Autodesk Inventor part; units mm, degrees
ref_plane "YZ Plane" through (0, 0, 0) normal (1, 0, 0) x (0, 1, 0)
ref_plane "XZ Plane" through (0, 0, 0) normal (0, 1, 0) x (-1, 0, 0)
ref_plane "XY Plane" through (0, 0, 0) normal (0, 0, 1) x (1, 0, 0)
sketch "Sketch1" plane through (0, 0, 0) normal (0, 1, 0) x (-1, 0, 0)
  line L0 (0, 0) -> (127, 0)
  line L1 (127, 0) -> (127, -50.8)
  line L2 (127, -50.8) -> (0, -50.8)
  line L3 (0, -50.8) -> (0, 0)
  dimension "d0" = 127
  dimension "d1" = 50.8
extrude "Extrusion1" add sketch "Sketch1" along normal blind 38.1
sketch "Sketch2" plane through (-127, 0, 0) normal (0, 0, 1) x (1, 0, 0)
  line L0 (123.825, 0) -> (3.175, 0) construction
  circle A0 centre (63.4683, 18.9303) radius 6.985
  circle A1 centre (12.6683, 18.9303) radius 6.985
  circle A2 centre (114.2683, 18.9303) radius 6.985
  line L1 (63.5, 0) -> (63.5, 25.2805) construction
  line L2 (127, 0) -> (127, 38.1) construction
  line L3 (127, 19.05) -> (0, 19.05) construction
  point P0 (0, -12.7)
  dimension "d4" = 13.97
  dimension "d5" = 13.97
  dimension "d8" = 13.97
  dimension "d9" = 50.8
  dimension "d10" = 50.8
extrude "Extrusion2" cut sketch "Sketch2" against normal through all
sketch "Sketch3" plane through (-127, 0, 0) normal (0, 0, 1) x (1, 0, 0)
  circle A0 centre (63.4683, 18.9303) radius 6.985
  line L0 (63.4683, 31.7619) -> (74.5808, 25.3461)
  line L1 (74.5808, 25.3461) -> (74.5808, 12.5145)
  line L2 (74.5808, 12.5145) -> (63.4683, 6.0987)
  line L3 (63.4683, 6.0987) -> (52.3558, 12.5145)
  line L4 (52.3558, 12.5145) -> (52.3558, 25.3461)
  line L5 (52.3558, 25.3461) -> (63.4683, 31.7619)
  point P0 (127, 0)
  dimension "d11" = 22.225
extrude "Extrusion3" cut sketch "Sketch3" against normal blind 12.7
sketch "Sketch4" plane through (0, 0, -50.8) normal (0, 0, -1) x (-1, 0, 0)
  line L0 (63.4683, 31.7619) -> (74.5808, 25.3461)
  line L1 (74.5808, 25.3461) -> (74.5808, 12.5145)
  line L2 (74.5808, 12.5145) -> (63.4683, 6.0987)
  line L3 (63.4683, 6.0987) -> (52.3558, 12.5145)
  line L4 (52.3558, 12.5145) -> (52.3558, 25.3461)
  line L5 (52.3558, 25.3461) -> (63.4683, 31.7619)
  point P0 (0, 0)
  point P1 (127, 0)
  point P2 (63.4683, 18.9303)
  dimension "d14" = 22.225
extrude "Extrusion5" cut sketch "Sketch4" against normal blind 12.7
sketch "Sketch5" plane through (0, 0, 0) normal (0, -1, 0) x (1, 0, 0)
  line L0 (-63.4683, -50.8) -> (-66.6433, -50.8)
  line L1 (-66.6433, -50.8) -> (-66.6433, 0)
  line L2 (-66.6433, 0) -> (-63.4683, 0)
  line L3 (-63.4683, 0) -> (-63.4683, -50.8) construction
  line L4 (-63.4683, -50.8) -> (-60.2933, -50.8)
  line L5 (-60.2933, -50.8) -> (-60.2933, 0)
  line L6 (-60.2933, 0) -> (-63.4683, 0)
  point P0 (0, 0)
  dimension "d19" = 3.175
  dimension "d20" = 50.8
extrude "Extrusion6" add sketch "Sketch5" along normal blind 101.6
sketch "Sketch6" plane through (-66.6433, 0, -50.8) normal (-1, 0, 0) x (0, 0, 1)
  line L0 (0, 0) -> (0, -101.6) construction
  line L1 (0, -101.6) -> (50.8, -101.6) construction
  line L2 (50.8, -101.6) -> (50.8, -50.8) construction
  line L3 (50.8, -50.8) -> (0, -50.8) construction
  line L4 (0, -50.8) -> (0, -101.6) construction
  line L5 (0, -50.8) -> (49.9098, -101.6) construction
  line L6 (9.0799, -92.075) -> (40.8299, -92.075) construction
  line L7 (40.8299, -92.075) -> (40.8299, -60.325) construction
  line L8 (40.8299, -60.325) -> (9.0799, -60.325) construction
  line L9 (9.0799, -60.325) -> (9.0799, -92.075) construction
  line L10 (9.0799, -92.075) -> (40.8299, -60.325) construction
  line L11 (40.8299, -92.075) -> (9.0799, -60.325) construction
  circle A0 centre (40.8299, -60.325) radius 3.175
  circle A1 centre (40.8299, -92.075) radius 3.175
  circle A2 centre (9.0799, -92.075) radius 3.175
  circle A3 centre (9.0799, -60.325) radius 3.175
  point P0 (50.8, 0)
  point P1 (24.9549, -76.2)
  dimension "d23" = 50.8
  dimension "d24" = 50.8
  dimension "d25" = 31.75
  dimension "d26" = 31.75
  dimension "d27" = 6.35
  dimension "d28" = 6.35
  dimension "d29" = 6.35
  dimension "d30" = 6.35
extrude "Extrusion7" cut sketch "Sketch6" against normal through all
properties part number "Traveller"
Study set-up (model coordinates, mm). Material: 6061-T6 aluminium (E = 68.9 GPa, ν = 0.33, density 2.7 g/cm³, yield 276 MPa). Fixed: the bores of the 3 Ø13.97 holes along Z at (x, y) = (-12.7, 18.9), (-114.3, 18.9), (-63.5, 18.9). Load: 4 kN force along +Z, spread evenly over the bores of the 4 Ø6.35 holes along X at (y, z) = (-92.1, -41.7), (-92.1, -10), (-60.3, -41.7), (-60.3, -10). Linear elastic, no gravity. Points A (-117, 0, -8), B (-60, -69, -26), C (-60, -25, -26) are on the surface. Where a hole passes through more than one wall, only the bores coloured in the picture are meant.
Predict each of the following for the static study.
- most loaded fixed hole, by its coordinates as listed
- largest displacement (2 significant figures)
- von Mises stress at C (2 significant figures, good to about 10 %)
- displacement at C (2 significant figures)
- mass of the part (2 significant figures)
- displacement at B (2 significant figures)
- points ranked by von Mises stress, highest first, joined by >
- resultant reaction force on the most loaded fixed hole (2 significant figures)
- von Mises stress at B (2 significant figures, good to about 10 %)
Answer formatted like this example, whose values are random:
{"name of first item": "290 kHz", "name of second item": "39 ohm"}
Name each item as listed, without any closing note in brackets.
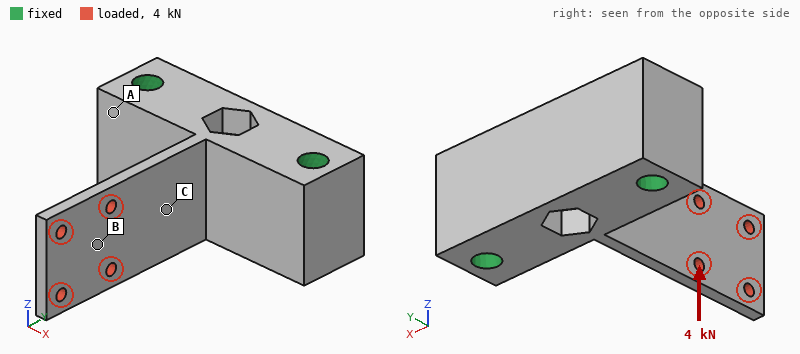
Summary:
{"most loaded fixed hole, by its coordinates as listed": "(-63.5, 18.9)", "largest displacement": "0.38 mm", "von Mises stress at C": "33 MPa", "displacement at C": "0.072 mm", "mass of the part": "670 g", "displacement at B": "0.24 mm", "points ranked by von Mises stress, highest first, joined by >": "C > B > A", "resultant reaction force on the most loaded fixed hole": "4.1 kN", "von Mises stress at B": "19 MPa"}
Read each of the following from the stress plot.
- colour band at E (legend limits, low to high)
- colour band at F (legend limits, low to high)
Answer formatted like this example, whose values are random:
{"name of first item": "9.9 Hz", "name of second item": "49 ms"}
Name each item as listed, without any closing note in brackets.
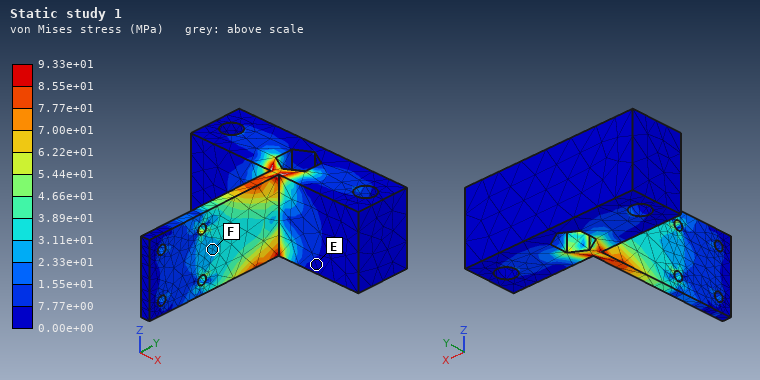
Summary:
{"colour band at E": "0.00e+00 to 7.77e+00 MPa", "colour band at F": "2.33e+01 to 3.11e+01 MPa"}
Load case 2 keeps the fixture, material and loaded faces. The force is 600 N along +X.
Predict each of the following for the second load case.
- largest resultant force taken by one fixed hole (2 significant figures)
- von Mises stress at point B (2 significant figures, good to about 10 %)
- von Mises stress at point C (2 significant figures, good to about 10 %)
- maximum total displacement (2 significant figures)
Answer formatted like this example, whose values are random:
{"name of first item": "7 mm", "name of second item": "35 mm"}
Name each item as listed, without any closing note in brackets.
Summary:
{"largest resultant force taken by one fixed hole": "730 N", "von Mises stress at point B": "23 MPa", "von Mises stress at point C": "82 MPa", "maximum total displacement": "1.9 mm"}
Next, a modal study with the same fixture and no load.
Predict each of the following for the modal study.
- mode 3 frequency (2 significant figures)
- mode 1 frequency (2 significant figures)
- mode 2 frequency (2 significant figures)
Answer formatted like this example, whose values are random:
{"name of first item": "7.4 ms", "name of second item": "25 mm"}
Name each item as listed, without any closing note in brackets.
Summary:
{"mode 3 frequency": "2700 Hz", "mode 1 frequency": "500 Hz", "mode 2 frequency": "2100 Hz"}
